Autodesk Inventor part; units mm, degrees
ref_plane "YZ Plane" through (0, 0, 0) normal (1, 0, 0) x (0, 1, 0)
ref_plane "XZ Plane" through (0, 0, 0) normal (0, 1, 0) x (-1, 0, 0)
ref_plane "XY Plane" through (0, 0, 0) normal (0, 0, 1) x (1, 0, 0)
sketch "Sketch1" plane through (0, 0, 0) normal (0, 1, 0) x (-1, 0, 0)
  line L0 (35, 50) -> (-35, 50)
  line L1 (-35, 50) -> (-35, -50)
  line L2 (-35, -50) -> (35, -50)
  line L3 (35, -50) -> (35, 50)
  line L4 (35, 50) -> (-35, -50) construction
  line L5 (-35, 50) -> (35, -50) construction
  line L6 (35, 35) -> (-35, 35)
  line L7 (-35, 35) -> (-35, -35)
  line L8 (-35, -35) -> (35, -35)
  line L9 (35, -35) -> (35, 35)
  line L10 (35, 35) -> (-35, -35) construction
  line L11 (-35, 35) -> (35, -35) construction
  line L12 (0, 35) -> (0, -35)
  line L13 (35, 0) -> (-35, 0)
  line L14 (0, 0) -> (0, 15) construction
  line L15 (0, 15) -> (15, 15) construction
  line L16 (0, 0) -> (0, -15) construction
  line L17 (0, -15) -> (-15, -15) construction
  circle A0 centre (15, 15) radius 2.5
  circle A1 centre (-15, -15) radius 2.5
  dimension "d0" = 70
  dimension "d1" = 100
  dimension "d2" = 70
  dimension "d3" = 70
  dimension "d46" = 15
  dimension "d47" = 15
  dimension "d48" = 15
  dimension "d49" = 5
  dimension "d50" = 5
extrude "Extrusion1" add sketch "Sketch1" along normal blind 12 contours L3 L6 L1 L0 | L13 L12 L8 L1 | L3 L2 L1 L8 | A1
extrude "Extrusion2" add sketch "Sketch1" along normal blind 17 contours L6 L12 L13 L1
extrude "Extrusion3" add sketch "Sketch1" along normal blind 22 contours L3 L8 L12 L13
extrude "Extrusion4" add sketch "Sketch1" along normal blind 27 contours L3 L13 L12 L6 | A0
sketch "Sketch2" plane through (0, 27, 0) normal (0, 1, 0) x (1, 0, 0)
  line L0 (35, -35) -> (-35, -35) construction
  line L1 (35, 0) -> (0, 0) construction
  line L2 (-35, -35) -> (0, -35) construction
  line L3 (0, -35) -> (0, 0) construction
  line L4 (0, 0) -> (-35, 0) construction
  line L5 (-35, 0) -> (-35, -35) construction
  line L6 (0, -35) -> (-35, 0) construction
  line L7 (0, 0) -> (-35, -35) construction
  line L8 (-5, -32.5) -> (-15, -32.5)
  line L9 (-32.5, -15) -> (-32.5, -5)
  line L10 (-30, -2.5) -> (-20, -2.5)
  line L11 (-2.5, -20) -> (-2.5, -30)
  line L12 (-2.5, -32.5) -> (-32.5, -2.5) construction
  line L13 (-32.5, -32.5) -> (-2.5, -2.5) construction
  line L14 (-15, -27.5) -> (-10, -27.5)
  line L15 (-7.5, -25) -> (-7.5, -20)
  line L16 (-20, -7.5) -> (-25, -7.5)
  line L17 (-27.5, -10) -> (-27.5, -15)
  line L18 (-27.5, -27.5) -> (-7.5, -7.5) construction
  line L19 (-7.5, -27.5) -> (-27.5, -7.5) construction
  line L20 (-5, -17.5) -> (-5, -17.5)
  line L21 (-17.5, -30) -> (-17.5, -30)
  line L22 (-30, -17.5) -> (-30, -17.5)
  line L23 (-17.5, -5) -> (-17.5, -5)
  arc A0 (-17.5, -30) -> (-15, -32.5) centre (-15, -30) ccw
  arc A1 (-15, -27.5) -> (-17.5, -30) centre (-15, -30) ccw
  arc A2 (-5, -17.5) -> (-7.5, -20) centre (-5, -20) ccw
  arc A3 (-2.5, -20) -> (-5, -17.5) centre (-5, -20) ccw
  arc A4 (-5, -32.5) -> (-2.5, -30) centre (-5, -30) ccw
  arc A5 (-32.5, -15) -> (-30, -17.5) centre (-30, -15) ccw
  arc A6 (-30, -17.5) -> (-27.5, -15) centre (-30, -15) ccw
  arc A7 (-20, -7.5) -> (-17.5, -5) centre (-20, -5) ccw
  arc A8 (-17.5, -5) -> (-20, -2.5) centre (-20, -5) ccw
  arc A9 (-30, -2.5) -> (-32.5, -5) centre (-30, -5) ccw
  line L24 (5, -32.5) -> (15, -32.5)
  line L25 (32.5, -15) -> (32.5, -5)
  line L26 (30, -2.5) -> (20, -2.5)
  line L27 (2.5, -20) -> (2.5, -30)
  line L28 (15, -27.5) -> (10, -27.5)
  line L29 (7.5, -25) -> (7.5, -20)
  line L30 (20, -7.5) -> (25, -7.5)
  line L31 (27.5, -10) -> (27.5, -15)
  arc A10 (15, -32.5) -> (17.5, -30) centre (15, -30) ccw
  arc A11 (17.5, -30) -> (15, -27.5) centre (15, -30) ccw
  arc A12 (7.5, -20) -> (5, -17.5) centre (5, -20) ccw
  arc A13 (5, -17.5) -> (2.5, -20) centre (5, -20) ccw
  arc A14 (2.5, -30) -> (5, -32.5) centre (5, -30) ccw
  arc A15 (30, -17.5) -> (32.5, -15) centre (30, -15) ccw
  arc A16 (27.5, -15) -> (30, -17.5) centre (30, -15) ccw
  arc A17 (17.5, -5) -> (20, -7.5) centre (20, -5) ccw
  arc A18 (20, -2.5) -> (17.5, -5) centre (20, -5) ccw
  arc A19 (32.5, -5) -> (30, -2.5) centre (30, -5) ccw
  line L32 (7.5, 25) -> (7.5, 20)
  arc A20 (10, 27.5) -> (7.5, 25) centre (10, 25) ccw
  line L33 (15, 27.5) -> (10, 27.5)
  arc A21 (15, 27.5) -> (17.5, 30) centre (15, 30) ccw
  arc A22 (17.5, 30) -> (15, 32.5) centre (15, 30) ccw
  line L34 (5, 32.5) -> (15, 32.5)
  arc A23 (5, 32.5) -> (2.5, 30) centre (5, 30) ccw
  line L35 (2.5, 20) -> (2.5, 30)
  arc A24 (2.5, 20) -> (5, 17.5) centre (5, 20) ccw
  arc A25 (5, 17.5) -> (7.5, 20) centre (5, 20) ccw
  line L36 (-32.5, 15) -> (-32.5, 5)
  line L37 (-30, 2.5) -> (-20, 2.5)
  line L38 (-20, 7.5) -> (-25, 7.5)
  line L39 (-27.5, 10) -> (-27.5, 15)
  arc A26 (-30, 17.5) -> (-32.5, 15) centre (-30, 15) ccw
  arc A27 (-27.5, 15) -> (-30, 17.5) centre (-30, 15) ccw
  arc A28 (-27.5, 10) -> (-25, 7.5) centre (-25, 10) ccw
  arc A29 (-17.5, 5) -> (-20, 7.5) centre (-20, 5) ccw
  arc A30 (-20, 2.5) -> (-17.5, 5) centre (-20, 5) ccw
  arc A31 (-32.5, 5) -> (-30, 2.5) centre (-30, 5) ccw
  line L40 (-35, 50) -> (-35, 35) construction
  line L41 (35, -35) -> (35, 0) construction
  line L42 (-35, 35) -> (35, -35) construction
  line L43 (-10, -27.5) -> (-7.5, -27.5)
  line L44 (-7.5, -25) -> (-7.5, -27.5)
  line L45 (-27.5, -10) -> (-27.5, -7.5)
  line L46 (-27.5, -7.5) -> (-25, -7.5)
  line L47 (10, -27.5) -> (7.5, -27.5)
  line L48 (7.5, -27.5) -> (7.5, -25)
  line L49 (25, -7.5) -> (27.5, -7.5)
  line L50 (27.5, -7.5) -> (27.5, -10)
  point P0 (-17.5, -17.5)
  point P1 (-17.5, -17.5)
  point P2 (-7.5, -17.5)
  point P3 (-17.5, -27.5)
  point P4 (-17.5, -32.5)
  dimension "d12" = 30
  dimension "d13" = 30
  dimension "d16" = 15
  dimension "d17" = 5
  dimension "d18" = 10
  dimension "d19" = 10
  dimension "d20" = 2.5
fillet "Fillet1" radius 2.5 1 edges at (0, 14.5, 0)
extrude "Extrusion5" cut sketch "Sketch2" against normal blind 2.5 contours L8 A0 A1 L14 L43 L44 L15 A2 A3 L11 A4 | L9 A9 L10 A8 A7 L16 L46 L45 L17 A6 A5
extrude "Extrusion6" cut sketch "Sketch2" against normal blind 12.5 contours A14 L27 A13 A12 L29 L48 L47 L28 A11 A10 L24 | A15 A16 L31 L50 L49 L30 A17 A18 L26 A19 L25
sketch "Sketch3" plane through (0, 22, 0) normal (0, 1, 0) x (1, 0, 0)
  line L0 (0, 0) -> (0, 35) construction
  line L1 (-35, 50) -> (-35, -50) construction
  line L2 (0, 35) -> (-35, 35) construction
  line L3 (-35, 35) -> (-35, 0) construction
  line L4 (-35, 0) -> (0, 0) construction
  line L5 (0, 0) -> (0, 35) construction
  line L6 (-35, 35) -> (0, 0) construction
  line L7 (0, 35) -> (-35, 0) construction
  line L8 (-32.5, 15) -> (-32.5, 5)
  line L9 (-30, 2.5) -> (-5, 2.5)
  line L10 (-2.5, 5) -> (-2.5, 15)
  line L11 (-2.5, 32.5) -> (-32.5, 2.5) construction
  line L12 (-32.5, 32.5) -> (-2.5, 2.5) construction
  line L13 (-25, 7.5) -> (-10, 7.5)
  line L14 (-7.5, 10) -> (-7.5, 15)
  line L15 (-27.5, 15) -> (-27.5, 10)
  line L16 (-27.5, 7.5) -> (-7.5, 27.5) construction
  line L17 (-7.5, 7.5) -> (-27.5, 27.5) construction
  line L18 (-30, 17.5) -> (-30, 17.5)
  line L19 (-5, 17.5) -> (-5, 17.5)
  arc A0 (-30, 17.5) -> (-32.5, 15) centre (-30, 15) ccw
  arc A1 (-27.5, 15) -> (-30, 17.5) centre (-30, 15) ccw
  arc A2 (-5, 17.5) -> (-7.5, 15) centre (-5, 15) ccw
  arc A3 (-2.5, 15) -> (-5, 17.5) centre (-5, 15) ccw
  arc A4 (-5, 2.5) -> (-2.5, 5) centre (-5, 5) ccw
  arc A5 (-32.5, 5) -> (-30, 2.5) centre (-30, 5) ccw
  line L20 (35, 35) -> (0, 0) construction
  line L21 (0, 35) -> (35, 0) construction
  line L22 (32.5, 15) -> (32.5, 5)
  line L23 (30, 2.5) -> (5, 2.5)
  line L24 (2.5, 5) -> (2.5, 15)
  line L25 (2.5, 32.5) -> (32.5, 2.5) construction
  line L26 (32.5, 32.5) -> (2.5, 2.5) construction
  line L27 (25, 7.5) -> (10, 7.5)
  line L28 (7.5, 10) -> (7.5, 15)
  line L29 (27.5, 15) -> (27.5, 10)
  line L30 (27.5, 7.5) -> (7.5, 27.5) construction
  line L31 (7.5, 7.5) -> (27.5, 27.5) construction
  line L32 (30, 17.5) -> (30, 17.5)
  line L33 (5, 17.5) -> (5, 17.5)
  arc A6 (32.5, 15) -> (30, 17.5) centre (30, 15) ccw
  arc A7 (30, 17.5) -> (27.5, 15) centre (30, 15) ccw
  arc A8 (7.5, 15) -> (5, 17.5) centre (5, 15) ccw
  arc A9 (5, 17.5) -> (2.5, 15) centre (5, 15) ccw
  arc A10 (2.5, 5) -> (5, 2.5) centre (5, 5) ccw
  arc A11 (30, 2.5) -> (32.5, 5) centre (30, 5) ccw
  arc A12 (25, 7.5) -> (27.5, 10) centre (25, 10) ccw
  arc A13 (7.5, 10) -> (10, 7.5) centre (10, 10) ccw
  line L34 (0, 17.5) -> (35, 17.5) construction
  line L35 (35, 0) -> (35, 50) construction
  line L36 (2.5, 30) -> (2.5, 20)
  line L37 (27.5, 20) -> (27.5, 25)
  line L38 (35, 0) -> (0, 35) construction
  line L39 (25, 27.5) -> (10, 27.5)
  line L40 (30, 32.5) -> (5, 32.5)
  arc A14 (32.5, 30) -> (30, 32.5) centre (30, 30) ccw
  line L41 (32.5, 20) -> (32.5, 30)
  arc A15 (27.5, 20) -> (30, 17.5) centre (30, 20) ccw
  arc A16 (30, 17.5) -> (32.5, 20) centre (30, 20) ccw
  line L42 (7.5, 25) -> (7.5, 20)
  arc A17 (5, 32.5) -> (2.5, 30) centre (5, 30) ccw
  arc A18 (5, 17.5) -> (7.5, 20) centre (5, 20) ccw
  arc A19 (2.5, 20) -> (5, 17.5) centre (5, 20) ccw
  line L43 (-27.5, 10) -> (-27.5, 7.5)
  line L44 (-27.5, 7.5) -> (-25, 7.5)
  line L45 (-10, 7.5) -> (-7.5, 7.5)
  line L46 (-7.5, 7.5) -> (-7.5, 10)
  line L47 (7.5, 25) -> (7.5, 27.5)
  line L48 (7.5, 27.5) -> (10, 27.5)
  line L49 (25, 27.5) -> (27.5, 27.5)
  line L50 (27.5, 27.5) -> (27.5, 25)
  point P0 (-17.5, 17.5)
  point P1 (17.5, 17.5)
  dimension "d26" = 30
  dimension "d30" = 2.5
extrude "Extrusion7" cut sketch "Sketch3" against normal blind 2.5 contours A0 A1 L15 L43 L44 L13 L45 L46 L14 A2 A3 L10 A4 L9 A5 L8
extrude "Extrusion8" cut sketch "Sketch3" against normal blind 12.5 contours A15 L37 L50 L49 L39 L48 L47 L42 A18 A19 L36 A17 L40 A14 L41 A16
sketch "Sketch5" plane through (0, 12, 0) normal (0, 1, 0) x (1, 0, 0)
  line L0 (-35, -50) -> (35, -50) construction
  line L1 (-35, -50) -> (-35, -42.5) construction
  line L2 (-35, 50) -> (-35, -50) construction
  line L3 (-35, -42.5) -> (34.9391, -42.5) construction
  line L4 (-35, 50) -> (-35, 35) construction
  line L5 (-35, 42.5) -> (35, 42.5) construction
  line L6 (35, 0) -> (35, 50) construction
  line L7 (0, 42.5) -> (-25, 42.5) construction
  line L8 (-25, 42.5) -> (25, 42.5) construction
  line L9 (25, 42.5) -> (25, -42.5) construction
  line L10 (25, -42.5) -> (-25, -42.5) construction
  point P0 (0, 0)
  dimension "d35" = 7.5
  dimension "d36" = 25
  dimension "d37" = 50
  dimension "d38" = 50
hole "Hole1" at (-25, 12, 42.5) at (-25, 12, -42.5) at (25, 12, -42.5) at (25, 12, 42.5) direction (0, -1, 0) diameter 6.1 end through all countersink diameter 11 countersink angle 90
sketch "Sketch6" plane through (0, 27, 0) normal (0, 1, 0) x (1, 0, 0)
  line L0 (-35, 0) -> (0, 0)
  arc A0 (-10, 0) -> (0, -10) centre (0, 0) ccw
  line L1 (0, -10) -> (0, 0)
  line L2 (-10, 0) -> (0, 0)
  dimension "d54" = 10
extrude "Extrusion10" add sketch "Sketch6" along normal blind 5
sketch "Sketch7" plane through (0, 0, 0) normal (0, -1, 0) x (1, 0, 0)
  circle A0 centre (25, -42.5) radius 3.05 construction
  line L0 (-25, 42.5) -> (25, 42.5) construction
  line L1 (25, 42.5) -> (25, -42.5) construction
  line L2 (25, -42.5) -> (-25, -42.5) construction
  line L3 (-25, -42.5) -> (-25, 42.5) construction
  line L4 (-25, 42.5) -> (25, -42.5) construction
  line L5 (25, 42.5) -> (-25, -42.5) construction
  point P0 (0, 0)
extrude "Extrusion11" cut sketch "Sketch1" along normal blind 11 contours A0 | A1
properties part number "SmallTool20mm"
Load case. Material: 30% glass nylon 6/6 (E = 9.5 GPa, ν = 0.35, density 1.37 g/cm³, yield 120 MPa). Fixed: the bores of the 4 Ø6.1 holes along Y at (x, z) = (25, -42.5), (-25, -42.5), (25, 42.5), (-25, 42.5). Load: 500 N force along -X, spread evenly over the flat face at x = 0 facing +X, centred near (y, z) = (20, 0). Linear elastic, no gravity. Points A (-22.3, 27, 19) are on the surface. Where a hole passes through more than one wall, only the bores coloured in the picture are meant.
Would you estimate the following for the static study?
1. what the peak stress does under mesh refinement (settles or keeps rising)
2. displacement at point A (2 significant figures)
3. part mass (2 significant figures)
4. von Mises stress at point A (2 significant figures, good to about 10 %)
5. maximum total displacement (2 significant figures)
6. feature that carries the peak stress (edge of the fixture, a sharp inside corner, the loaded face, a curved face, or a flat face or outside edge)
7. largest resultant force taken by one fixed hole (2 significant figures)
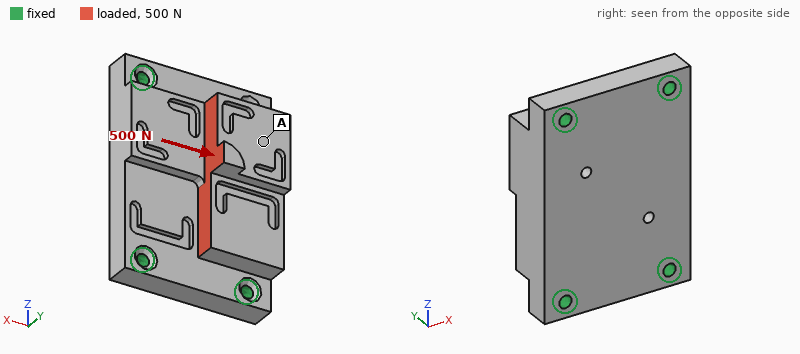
keeps rising
6.7 µm
160 g
0.37 MPa
12 µm
edge of the fixture
190 N
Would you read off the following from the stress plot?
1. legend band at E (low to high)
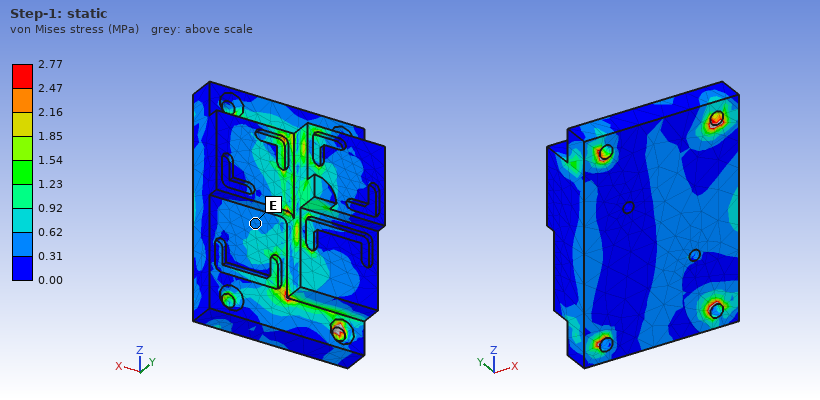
0.31 to 0.62 MPa
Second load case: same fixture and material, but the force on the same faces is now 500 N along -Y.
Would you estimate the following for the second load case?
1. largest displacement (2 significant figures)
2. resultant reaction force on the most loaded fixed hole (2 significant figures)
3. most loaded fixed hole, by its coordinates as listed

18 µm
180 N
(-25, -42.5)
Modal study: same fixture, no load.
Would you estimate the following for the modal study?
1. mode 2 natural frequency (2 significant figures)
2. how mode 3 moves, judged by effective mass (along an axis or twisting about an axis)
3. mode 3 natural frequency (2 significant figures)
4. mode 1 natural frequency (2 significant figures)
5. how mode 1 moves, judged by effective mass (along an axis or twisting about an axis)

4700 Hz
along X
6300 Hz
3500 Hz
along Y
